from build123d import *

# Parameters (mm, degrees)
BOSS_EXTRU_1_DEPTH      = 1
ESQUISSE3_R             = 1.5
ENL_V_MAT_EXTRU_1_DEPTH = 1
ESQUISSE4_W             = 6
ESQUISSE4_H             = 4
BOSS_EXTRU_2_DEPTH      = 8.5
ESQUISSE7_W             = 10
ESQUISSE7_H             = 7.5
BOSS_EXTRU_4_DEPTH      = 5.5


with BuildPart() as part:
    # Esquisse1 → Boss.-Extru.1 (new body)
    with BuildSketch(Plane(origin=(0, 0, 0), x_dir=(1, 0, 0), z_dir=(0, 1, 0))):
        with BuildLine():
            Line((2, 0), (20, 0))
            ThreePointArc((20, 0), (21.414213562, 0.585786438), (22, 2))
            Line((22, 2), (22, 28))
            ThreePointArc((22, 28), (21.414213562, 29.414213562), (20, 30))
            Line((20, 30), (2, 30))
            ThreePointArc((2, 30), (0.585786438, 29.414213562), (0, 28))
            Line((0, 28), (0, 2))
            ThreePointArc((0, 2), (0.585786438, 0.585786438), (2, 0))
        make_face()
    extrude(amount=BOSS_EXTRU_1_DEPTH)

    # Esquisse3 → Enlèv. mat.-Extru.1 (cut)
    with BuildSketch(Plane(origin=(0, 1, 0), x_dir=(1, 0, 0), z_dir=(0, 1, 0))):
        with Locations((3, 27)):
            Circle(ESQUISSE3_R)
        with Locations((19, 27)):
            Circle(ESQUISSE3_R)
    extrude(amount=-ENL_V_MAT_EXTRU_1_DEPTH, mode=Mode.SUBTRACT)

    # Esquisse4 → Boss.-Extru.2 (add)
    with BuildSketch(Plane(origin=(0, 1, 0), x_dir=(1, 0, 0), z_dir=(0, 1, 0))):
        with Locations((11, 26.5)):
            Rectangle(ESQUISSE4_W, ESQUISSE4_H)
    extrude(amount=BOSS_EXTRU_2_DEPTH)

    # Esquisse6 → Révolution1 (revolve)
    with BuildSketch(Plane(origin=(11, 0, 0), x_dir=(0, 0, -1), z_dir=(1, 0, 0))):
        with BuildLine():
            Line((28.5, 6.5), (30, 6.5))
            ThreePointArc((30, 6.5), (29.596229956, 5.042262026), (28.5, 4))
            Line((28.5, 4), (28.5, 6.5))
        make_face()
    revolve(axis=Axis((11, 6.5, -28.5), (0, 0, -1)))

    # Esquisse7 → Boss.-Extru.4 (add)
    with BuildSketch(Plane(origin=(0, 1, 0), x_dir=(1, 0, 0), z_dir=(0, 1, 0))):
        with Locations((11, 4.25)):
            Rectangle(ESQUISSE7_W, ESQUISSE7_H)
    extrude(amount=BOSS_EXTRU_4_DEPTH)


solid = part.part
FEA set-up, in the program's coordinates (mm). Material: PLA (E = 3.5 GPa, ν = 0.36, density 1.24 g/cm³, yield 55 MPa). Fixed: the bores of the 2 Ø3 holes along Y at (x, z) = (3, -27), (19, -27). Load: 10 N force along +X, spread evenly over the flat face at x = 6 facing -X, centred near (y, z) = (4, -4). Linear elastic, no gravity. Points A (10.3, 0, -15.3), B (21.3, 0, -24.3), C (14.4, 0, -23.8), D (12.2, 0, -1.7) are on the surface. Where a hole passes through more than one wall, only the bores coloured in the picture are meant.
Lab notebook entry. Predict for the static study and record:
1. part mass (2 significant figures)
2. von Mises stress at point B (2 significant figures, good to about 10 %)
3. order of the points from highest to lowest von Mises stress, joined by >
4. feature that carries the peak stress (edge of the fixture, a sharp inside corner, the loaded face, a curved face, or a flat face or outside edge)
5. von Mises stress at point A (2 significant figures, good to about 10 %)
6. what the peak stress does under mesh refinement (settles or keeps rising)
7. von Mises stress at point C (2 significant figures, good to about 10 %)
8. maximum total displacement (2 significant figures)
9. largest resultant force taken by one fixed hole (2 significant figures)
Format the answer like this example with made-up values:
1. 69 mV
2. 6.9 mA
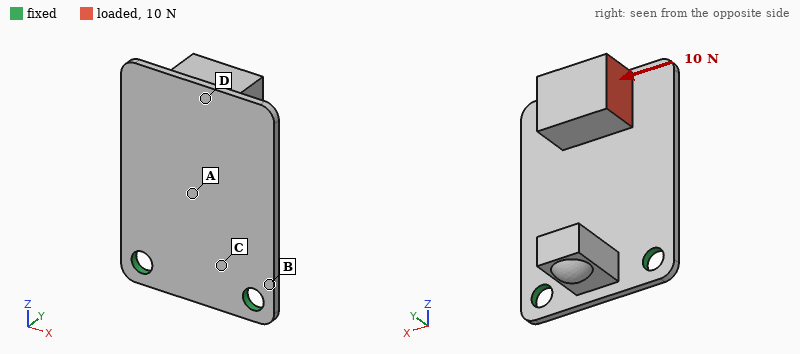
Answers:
1. 1.6 g
2. 9.2 MPa
3. B > A > C > D
4. edge of the fixture
5. 5.0 MPa
6. keeps rising
7. 3.3 MPa
8. 0.39 mm
9. 14 N
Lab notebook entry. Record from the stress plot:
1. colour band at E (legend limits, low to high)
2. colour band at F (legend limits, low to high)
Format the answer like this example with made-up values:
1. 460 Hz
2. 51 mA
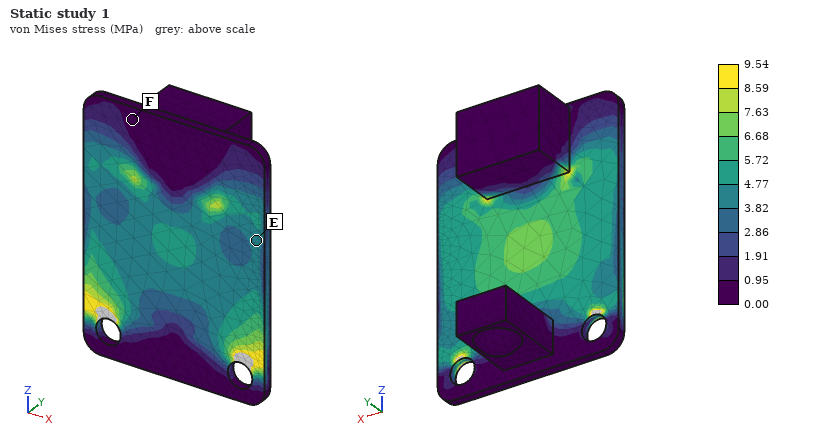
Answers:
1. 3.82 to 4.77 MPa
2. 0.00 to 0.95 MPa
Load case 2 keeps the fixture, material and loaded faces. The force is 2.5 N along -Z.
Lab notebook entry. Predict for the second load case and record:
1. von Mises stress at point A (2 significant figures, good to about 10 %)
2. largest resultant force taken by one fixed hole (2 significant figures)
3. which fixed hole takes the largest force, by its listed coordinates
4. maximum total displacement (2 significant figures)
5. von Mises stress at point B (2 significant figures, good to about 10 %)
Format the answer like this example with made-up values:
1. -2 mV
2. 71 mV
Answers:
1. 1.8 MPa
2. 2.0 N
3. (3, -27)
4. 0.40 mm
5. 2.2 MPa
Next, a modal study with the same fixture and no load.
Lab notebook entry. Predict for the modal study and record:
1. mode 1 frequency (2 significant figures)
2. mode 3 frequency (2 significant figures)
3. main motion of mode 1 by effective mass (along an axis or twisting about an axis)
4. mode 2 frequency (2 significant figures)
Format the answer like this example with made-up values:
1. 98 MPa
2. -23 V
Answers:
1. 240 Hz
2. 1700 Hz
3. along Y
4. 960 Hz
